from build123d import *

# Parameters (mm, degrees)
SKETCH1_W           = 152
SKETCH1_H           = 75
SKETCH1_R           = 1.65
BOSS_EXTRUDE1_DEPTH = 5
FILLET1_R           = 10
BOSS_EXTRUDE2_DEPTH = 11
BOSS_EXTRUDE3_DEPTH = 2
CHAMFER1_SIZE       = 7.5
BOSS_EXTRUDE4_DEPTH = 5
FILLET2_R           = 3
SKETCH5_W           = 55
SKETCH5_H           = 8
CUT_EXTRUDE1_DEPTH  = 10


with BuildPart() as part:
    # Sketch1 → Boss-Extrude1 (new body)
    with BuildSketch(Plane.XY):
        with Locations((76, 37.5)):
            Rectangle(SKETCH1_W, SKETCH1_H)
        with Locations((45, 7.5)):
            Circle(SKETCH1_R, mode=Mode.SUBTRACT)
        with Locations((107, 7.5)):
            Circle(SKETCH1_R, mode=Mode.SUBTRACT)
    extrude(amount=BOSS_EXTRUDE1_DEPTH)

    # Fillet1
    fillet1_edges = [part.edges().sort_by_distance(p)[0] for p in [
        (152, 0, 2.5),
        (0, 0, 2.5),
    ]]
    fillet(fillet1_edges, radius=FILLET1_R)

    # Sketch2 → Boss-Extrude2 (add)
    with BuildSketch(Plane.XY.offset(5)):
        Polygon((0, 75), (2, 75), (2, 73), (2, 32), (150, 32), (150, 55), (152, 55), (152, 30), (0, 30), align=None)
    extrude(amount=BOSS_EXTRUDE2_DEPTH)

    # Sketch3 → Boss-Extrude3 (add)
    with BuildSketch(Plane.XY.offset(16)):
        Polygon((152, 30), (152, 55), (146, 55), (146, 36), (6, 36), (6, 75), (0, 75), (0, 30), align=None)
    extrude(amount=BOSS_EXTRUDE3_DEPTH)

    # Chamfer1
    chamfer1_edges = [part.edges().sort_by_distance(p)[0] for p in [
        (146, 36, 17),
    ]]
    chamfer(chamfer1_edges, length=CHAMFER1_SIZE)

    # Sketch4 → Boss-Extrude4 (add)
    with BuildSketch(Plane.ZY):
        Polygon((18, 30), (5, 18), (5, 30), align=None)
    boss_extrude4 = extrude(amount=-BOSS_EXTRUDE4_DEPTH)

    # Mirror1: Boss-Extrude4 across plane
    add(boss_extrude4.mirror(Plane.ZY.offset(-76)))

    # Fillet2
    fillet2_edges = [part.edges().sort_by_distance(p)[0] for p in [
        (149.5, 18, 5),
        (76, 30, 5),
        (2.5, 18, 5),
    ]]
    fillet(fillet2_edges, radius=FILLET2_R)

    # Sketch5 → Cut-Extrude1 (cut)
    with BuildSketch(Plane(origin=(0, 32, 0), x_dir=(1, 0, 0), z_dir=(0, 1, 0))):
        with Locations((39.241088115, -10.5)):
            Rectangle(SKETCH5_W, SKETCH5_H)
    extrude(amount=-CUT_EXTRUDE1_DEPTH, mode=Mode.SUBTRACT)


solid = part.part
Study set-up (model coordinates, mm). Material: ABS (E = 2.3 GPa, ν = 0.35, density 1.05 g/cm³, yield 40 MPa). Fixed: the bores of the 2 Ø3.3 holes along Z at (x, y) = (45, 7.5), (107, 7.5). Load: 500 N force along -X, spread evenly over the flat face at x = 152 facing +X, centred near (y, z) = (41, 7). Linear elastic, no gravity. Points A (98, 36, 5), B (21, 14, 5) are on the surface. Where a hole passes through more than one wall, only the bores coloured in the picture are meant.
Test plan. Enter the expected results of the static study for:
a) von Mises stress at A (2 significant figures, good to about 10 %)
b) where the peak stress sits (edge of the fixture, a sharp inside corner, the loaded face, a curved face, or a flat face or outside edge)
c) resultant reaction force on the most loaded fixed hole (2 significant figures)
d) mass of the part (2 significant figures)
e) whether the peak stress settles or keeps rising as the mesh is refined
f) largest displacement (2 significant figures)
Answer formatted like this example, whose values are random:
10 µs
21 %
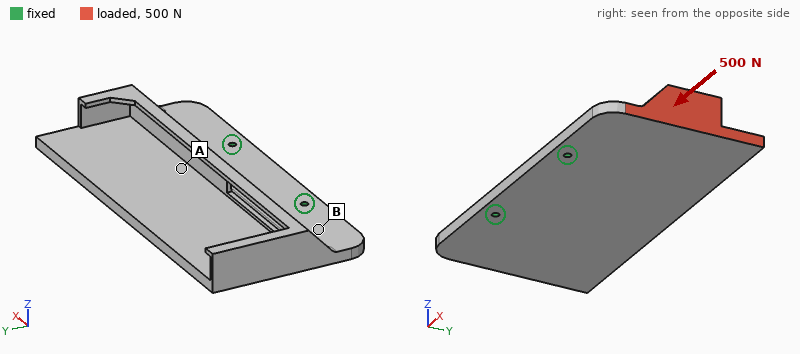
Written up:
3.0 MPa
edge of the fixture
380 N
67 g
keeps rising
1.2 mm
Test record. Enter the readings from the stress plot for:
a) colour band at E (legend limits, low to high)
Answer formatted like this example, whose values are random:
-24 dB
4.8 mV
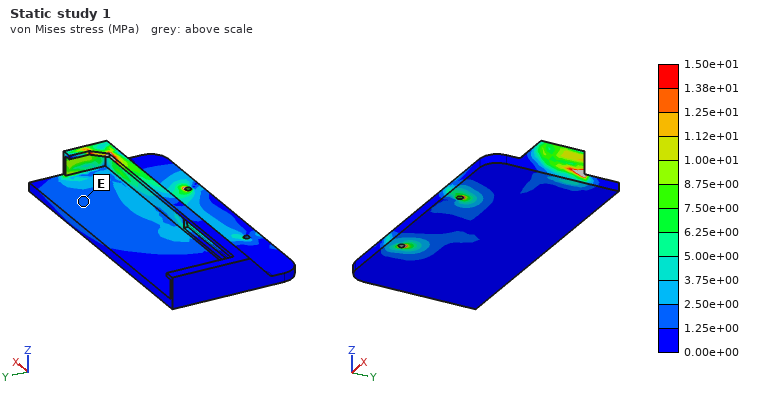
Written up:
1.25e+00 to 2.50e+00 MPa
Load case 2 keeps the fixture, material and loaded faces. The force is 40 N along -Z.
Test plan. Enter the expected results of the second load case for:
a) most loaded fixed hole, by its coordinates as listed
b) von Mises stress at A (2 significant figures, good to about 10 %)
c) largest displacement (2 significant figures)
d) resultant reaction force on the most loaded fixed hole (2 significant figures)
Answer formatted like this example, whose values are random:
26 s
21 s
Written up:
(107, 7.5)
1.9 MPa
2.0 mm
64 N
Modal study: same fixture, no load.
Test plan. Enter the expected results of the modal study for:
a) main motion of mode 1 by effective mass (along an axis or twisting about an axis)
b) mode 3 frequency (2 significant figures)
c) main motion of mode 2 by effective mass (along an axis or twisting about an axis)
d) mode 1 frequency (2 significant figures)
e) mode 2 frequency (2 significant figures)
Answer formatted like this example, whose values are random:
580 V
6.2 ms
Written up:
along Z
540 Hz
twisting about Y
180 Hz
240 Hz
